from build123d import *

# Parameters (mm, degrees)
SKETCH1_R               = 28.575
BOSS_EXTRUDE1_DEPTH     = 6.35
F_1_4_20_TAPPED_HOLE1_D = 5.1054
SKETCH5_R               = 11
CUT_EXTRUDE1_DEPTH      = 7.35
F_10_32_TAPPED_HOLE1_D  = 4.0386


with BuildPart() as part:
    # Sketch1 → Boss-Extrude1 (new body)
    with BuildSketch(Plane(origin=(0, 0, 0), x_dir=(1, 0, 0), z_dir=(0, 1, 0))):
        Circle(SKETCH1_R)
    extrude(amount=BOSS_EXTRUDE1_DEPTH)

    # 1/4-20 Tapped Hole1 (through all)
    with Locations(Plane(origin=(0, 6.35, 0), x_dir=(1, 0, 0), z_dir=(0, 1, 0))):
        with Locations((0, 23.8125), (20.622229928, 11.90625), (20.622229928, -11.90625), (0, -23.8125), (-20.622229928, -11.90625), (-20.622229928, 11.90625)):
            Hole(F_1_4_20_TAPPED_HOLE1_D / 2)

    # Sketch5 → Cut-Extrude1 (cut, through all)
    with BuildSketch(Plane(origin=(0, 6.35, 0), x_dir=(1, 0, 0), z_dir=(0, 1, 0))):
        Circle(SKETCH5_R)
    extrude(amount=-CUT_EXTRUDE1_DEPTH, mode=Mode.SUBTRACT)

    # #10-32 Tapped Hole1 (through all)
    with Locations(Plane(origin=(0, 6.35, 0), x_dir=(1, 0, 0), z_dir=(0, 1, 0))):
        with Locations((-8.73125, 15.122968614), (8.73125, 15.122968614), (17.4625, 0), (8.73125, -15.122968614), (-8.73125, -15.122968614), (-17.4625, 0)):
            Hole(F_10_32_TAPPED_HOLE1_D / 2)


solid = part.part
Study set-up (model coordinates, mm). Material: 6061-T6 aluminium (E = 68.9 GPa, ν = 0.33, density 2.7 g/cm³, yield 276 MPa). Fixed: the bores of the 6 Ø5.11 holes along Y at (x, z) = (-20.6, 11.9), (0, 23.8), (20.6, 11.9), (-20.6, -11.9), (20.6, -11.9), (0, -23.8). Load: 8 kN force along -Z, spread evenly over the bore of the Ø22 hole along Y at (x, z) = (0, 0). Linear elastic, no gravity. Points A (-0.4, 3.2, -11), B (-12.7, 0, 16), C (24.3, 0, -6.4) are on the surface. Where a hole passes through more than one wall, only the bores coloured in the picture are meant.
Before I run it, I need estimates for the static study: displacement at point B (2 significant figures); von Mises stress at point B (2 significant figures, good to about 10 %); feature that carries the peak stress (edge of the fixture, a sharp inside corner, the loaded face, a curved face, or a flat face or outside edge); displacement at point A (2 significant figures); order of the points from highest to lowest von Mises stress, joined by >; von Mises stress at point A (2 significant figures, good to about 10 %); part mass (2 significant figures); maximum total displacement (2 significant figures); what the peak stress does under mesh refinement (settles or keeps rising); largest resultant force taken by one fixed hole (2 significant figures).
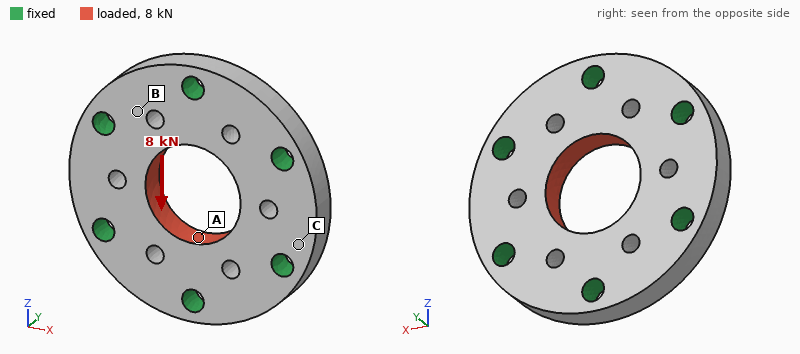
2.4 µm
8.8 MPa
edge of the fixture
3.9 µm
A > B > C
19 MPa
34 g
5.1 µm
keeps rising
1.9 kN
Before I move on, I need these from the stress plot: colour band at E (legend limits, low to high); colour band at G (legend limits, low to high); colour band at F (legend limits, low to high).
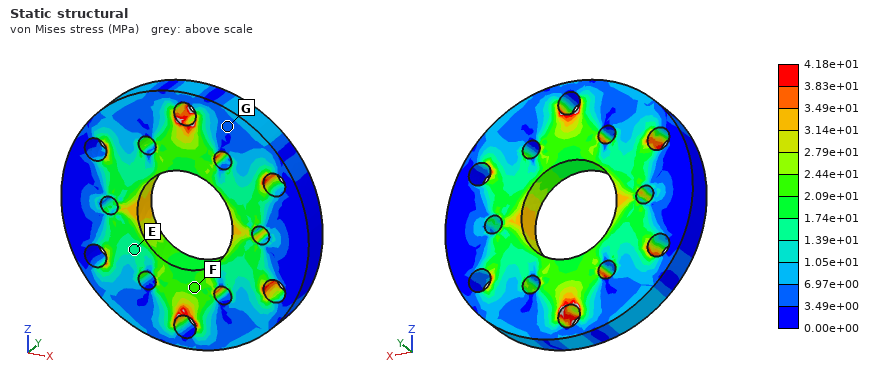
1.39e+01 to 1.74e+01 MPa
3.49e+00 to 6.97e+00 MPa
2.09e+01 to 2.44e+01 MPa
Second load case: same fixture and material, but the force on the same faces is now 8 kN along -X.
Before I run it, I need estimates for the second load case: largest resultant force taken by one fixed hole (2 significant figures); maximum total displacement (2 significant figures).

1.7 kN
5.2 µm
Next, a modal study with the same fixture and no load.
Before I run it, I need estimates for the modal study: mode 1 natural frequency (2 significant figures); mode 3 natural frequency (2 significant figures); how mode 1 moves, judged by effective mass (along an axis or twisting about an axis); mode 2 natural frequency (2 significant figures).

32 kHz
39 kHz
along Y
39 kHz
